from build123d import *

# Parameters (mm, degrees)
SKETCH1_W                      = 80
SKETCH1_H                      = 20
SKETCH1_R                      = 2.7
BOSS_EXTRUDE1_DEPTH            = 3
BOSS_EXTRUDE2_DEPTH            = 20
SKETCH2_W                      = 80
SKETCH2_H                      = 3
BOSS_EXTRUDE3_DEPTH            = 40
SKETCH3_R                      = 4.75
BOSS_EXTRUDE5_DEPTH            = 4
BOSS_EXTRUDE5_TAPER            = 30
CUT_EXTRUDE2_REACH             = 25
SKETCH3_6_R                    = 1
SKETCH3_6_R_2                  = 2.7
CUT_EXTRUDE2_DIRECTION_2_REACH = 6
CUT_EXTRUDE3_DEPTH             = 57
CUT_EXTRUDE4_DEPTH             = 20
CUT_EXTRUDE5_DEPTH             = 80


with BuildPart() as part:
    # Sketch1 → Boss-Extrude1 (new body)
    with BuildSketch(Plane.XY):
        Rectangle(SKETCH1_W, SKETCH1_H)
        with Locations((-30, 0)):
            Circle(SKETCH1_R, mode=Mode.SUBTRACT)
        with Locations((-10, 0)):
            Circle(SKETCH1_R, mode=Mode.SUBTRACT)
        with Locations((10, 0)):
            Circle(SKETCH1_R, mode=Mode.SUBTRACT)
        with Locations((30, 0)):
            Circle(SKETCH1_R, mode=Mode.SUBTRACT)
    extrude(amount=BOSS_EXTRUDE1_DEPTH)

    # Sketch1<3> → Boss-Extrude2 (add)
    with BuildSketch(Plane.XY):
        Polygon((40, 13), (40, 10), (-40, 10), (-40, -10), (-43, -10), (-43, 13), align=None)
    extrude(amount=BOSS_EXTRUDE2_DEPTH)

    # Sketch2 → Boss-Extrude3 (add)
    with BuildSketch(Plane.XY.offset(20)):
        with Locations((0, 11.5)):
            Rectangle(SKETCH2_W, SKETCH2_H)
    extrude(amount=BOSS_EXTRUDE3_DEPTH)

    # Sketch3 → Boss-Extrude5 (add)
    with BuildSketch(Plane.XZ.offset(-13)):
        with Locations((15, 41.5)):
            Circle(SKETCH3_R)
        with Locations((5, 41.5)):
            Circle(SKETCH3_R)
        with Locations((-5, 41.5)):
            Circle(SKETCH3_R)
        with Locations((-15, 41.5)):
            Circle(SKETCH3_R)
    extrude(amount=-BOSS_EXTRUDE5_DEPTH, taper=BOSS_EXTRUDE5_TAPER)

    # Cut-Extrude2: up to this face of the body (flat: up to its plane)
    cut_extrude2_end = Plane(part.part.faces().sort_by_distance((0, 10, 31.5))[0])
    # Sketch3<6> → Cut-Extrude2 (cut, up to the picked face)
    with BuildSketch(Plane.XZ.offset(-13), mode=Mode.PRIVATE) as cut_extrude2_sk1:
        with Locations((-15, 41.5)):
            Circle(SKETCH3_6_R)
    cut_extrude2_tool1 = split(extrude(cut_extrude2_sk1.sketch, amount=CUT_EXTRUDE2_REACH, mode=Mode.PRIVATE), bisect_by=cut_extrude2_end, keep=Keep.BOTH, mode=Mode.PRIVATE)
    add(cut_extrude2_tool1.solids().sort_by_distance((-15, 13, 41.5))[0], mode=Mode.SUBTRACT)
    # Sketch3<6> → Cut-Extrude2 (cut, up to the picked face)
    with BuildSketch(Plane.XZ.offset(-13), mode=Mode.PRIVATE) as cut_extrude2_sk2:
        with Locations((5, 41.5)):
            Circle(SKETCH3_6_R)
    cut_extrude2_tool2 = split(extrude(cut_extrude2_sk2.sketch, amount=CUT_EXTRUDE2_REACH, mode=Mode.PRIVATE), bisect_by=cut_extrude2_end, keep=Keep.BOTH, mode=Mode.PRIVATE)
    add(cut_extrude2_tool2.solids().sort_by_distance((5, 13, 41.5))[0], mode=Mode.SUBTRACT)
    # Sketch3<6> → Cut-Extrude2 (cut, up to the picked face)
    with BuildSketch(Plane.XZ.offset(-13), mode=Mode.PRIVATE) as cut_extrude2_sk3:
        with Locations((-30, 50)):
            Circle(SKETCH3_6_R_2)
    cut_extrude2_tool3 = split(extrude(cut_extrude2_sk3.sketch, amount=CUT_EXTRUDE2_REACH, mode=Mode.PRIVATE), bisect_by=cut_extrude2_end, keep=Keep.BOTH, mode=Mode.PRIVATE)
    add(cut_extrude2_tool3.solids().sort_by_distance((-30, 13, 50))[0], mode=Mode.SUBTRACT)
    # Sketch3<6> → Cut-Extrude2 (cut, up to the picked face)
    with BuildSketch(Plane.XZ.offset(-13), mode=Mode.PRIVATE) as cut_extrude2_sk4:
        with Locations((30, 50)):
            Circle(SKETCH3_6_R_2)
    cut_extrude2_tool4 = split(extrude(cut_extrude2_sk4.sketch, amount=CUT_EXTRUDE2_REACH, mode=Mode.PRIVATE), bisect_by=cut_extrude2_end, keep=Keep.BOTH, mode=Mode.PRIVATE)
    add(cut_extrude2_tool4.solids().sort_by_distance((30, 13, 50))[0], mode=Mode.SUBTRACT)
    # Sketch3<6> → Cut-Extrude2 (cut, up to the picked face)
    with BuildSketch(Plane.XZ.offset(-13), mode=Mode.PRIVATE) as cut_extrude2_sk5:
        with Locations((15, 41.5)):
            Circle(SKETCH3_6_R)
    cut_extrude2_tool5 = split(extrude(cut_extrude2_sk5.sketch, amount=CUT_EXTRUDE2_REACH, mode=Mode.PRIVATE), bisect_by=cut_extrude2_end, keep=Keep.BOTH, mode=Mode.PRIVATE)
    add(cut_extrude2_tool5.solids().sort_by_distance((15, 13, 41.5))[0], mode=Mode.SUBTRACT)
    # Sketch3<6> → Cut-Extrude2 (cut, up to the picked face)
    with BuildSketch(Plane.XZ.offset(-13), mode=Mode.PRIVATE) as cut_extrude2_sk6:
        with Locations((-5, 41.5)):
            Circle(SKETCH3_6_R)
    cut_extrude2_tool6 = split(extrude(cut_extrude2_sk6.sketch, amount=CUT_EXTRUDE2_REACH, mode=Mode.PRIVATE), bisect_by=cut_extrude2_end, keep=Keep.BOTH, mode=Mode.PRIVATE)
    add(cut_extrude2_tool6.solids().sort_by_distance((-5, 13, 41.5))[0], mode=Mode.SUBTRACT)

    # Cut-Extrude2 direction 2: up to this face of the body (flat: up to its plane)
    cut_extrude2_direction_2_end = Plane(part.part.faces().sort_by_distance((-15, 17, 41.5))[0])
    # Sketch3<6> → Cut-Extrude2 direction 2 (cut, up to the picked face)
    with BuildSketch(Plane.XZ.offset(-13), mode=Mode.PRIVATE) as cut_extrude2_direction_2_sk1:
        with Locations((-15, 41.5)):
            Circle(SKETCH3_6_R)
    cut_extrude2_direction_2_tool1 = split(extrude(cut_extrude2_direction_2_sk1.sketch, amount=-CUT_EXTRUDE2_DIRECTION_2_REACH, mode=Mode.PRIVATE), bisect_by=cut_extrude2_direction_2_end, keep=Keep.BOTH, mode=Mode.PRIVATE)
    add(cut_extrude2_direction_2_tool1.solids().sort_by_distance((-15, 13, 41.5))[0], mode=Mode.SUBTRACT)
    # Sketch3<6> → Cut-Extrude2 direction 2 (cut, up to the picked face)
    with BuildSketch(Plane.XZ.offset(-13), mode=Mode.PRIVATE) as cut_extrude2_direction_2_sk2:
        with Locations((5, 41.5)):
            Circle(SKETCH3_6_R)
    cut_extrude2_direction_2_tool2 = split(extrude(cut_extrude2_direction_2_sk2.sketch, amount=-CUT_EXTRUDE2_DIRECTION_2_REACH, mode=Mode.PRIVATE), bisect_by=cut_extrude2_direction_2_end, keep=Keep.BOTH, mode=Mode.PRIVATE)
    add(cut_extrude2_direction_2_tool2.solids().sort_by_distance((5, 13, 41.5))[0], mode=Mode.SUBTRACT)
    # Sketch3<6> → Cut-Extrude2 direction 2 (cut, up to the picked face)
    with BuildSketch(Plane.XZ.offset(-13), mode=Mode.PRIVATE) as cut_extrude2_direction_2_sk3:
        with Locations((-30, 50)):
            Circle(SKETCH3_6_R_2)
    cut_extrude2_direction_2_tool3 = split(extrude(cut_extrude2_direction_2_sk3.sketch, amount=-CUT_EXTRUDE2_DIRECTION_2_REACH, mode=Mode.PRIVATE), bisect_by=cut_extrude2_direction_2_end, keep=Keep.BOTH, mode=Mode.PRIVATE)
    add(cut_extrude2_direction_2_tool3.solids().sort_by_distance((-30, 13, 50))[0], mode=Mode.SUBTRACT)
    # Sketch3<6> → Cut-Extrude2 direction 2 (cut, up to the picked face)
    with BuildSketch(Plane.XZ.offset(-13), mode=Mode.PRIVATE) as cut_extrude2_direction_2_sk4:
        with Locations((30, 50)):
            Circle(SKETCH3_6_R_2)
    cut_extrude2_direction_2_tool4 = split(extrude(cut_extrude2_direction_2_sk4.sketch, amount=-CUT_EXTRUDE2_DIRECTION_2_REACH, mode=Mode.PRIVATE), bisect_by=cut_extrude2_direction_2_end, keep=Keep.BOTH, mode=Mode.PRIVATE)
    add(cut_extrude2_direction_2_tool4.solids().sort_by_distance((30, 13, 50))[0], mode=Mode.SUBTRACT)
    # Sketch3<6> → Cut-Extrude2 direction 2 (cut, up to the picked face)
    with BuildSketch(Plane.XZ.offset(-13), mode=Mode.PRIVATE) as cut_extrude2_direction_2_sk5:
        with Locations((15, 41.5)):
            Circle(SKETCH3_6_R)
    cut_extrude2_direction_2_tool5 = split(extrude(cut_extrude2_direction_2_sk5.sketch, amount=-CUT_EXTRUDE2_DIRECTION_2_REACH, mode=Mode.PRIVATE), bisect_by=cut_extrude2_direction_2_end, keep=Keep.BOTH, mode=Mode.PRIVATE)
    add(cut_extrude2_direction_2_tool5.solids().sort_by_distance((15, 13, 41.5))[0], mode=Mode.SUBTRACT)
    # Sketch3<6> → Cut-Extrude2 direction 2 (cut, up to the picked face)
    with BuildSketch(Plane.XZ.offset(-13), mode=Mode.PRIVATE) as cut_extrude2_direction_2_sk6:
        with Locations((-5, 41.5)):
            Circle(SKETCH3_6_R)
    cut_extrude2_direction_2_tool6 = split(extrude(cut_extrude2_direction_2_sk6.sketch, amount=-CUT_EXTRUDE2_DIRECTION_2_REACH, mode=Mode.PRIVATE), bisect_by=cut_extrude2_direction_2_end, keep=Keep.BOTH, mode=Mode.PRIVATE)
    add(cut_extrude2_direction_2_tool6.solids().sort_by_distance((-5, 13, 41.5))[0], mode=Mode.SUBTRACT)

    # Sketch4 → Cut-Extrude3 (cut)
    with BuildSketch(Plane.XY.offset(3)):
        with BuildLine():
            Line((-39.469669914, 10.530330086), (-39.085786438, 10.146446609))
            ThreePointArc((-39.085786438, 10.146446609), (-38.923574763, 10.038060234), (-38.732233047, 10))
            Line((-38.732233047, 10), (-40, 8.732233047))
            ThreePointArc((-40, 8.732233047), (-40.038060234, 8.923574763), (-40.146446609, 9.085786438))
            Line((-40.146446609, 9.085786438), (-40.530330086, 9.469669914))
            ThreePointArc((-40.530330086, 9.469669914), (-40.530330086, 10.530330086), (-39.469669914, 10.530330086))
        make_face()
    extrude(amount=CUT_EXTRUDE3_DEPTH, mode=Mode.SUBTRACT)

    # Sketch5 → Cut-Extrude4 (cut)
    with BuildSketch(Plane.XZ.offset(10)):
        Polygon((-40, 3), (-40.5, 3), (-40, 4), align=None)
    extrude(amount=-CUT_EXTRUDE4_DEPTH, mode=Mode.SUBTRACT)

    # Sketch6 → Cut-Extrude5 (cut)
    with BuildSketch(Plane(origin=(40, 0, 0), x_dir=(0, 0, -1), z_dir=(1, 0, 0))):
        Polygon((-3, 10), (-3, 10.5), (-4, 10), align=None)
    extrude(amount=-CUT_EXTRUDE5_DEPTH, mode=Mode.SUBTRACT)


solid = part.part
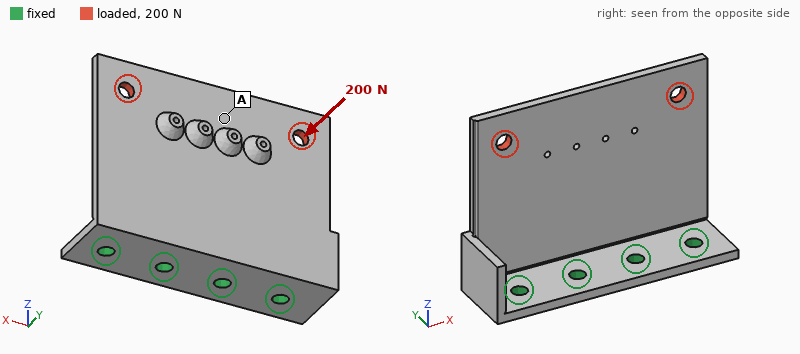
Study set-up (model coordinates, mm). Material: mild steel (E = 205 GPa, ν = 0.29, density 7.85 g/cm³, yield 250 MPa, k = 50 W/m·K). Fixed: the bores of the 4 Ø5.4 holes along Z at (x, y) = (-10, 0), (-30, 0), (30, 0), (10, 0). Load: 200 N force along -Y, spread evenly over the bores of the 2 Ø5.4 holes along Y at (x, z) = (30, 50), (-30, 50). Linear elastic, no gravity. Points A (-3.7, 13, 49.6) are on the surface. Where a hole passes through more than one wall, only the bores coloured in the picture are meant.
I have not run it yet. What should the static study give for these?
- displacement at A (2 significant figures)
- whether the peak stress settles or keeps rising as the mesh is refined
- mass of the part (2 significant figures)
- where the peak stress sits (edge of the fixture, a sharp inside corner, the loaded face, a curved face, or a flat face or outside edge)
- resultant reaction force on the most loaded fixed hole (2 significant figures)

0.25 mm
keeps rising
160 g
a sharp inside corner
70 N
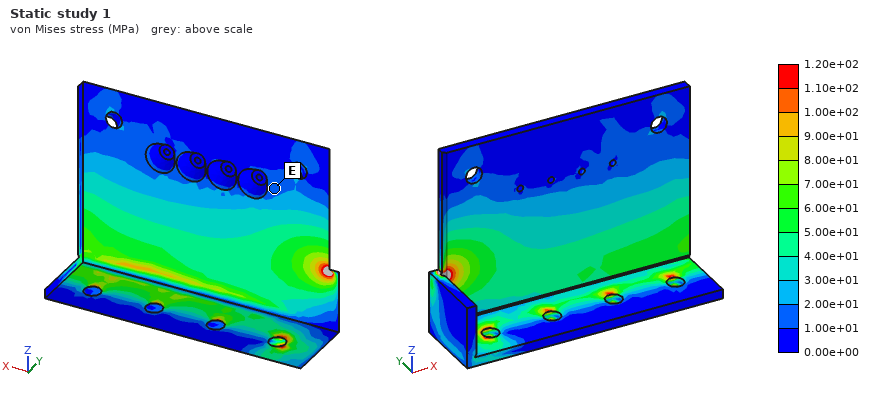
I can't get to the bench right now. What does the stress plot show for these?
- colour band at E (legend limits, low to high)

1.00e+01 to 2.00e+01 MPa
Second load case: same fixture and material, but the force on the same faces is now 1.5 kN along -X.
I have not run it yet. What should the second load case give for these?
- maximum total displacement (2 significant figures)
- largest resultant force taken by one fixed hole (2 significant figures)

0.12 mm
1.2 kN
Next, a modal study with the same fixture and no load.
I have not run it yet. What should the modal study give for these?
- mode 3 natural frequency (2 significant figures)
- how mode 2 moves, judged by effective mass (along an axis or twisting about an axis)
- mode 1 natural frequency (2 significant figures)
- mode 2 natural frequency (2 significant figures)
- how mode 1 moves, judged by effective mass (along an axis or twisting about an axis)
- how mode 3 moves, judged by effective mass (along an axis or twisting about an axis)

3100 Hz
twisting about Z
610 Hz
1500 Hz
along Y
along X
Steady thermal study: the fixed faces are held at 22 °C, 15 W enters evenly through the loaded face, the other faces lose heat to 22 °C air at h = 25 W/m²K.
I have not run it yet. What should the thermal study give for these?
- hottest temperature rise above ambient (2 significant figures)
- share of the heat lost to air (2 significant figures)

60 K
49 %
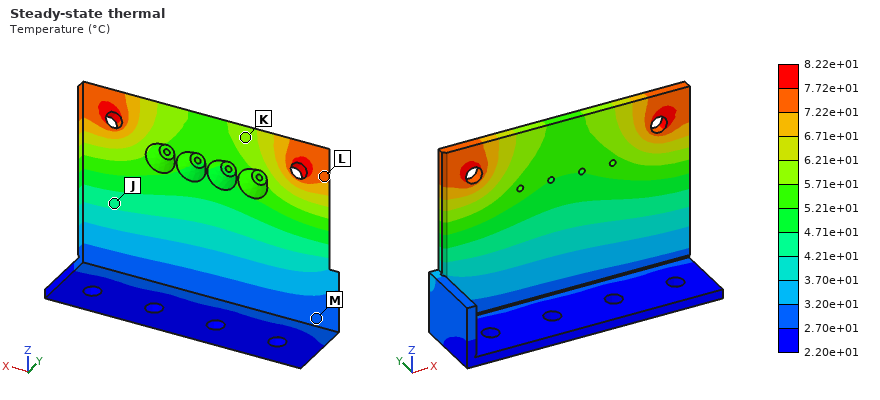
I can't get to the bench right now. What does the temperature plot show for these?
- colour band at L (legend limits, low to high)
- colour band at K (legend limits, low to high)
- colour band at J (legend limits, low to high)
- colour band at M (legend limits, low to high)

7.22e+01 to 7.72e+01 °C
5.71e+01 to 6.21e+01 °C
4.21e+01 to 4.71e+01 °C
2.70e+01 to 3.20e+01 °C
